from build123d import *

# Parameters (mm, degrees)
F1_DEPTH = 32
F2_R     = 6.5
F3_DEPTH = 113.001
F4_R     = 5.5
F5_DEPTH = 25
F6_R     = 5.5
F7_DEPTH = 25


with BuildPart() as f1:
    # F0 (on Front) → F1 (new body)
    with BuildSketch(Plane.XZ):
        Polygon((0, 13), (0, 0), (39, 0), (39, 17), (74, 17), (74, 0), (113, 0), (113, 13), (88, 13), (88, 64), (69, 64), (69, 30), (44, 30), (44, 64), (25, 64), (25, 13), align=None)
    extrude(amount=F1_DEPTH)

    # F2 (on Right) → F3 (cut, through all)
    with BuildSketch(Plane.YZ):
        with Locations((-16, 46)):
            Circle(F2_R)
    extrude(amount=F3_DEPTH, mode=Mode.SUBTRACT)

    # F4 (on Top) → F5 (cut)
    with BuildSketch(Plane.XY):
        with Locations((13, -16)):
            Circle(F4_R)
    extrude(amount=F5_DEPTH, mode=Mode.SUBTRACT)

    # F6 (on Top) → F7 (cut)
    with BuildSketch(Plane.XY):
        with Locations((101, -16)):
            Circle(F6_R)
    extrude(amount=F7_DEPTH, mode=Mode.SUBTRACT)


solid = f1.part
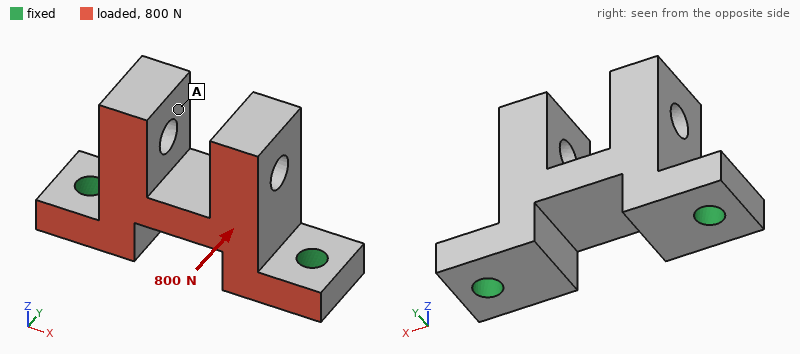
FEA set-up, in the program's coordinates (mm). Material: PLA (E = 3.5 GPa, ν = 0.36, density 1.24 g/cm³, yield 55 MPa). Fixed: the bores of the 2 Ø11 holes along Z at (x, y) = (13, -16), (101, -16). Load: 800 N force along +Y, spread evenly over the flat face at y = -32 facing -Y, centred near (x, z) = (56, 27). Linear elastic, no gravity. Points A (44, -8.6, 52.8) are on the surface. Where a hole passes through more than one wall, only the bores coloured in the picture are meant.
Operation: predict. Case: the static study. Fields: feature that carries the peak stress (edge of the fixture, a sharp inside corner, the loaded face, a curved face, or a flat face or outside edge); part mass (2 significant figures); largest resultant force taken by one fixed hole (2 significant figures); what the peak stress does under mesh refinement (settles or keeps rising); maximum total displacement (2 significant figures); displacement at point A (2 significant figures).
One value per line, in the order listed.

edge of the fixture
120 g
410 N
keeps rising
0.33 mm
0.26 mm
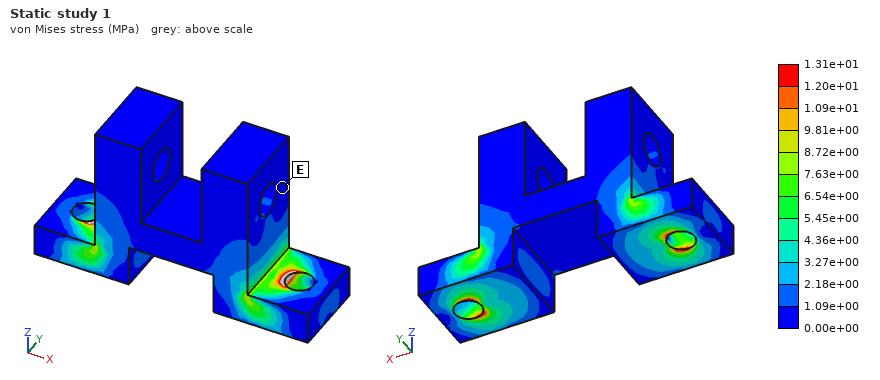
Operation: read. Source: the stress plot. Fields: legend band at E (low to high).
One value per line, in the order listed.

0.00e+00 to 1.09e+00 MPa
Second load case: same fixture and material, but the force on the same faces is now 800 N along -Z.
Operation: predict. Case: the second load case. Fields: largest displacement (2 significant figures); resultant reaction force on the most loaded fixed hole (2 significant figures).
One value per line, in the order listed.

0.21 mm
450 N
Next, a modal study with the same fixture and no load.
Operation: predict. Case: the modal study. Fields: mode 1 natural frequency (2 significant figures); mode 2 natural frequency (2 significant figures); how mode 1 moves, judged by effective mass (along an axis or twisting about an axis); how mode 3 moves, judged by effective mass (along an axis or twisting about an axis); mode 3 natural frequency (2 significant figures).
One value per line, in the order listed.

890 Hz
1500 Hz
along Y
along X
1800 Hz
